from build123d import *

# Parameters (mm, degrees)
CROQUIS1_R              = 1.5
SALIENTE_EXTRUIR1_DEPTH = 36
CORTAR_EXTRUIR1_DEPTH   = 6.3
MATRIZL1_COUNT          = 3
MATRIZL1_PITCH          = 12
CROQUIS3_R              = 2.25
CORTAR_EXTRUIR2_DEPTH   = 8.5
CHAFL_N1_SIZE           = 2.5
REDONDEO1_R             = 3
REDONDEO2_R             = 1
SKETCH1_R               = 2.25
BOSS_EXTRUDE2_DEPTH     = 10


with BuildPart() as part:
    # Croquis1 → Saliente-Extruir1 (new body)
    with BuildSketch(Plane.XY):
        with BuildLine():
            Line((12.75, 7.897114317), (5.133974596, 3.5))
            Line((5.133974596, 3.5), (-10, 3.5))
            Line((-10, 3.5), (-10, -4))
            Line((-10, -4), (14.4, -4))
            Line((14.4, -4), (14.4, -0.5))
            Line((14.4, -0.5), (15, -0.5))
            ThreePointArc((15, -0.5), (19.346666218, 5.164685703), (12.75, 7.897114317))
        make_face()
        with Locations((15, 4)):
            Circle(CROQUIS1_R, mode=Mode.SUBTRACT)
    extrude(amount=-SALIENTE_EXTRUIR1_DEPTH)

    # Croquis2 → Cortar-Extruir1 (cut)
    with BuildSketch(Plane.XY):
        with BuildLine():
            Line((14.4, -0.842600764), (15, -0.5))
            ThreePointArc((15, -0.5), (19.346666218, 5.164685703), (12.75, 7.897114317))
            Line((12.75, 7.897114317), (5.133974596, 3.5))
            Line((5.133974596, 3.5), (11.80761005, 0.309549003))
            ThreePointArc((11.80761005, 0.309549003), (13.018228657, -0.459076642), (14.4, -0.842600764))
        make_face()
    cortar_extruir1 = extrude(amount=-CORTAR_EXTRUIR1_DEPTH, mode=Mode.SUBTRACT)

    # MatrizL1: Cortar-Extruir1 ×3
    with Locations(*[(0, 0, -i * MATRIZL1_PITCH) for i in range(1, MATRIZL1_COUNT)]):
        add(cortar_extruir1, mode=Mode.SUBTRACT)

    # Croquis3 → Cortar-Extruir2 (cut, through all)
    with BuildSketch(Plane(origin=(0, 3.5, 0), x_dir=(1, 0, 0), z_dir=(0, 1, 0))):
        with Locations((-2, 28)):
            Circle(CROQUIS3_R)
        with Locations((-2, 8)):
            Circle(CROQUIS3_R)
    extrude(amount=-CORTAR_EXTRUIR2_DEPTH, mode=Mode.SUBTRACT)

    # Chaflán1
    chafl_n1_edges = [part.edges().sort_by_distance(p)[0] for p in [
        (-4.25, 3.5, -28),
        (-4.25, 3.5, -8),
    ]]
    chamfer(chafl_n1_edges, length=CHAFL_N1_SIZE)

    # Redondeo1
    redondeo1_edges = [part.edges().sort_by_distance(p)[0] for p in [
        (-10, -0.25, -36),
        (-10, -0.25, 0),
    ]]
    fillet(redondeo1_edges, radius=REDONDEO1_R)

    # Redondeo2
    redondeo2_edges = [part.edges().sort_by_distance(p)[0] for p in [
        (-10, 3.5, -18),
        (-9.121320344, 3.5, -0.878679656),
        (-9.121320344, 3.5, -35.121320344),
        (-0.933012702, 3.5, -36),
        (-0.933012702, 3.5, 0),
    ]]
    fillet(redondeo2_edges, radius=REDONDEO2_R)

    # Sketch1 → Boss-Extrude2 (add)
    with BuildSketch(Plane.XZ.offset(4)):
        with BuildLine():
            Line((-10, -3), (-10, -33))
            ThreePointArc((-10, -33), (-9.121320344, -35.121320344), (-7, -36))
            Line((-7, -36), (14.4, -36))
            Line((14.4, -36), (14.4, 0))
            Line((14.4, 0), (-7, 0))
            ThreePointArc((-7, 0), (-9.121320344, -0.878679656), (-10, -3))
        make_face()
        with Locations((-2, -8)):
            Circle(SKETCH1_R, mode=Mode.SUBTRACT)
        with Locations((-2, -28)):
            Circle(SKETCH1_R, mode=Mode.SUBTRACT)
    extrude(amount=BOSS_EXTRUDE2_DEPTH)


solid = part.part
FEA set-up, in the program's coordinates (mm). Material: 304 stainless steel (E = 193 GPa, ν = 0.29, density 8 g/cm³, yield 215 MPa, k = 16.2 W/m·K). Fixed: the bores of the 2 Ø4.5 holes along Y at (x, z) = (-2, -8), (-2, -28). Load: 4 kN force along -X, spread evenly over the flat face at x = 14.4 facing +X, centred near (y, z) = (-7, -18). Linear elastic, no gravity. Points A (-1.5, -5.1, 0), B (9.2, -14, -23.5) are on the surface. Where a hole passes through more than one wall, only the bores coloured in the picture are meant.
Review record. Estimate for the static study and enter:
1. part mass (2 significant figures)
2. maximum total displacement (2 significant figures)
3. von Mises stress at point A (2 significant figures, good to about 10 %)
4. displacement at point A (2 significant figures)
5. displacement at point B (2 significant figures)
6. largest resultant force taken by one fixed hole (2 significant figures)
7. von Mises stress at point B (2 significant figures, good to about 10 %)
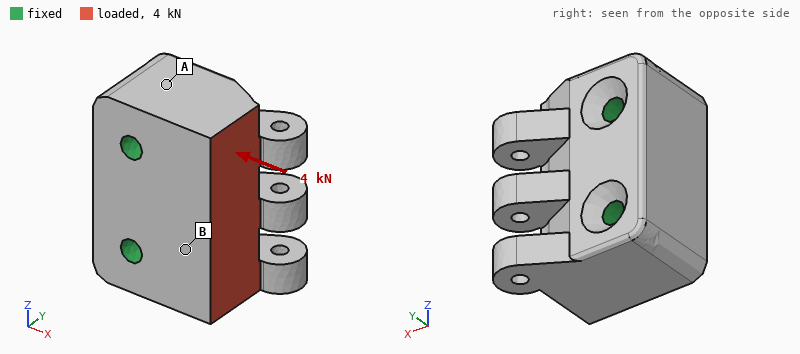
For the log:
120 g
1.1 µm
3.7 MPa
0.26 µm
0.73 µm
2.0 kN
9.1 MPa
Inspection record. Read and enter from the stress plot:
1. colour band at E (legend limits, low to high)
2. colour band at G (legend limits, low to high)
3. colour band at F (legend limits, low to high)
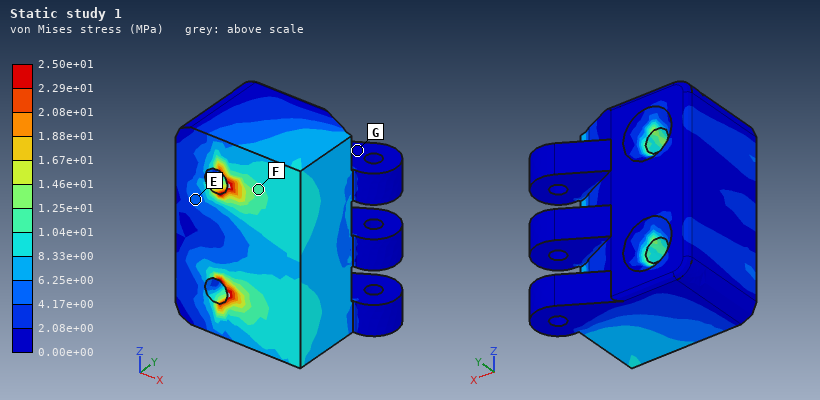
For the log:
4.17e+00 to 6.25e+00 MPa
0.00e+00 to 2.08e+00 MPa
1.04e+01 to 1.25e+01 MPa
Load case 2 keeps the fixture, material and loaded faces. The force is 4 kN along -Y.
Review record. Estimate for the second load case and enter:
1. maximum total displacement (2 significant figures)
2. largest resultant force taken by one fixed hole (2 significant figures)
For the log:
6.5 µm
2.0 kN
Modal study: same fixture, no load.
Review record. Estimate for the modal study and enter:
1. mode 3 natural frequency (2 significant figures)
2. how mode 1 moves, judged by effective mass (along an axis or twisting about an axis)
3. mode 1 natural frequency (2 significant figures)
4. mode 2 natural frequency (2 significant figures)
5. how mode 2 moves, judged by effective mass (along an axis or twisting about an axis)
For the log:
30 kHz
along Y
23 kHz
26 kHz
along Z
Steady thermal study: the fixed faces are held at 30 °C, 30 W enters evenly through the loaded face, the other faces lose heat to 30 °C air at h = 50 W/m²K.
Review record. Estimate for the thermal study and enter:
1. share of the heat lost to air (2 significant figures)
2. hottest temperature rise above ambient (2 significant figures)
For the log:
12 %
54 K
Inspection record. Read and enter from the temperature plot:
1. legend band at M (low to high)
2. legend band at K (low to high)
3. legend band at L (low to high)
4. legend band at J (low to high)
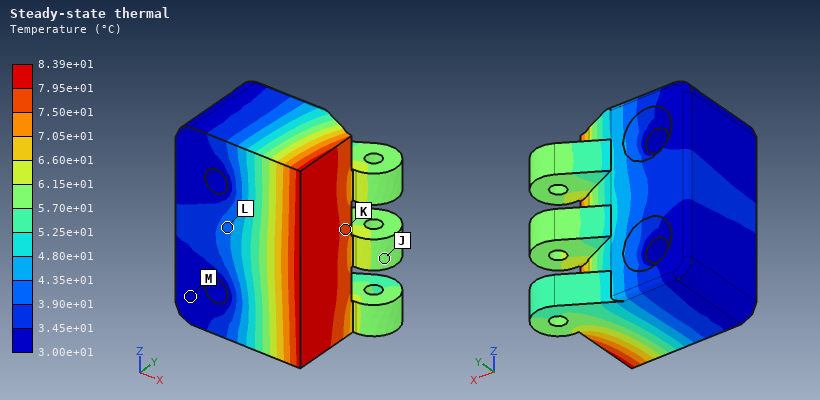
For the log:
3.00e+01 to 3.45e+01 °C
7.50e+01 to 7.95e+01 °C
3.90e+01 to 4.35e+01 °C
5.70e+01 to 6.15e+01 °C
